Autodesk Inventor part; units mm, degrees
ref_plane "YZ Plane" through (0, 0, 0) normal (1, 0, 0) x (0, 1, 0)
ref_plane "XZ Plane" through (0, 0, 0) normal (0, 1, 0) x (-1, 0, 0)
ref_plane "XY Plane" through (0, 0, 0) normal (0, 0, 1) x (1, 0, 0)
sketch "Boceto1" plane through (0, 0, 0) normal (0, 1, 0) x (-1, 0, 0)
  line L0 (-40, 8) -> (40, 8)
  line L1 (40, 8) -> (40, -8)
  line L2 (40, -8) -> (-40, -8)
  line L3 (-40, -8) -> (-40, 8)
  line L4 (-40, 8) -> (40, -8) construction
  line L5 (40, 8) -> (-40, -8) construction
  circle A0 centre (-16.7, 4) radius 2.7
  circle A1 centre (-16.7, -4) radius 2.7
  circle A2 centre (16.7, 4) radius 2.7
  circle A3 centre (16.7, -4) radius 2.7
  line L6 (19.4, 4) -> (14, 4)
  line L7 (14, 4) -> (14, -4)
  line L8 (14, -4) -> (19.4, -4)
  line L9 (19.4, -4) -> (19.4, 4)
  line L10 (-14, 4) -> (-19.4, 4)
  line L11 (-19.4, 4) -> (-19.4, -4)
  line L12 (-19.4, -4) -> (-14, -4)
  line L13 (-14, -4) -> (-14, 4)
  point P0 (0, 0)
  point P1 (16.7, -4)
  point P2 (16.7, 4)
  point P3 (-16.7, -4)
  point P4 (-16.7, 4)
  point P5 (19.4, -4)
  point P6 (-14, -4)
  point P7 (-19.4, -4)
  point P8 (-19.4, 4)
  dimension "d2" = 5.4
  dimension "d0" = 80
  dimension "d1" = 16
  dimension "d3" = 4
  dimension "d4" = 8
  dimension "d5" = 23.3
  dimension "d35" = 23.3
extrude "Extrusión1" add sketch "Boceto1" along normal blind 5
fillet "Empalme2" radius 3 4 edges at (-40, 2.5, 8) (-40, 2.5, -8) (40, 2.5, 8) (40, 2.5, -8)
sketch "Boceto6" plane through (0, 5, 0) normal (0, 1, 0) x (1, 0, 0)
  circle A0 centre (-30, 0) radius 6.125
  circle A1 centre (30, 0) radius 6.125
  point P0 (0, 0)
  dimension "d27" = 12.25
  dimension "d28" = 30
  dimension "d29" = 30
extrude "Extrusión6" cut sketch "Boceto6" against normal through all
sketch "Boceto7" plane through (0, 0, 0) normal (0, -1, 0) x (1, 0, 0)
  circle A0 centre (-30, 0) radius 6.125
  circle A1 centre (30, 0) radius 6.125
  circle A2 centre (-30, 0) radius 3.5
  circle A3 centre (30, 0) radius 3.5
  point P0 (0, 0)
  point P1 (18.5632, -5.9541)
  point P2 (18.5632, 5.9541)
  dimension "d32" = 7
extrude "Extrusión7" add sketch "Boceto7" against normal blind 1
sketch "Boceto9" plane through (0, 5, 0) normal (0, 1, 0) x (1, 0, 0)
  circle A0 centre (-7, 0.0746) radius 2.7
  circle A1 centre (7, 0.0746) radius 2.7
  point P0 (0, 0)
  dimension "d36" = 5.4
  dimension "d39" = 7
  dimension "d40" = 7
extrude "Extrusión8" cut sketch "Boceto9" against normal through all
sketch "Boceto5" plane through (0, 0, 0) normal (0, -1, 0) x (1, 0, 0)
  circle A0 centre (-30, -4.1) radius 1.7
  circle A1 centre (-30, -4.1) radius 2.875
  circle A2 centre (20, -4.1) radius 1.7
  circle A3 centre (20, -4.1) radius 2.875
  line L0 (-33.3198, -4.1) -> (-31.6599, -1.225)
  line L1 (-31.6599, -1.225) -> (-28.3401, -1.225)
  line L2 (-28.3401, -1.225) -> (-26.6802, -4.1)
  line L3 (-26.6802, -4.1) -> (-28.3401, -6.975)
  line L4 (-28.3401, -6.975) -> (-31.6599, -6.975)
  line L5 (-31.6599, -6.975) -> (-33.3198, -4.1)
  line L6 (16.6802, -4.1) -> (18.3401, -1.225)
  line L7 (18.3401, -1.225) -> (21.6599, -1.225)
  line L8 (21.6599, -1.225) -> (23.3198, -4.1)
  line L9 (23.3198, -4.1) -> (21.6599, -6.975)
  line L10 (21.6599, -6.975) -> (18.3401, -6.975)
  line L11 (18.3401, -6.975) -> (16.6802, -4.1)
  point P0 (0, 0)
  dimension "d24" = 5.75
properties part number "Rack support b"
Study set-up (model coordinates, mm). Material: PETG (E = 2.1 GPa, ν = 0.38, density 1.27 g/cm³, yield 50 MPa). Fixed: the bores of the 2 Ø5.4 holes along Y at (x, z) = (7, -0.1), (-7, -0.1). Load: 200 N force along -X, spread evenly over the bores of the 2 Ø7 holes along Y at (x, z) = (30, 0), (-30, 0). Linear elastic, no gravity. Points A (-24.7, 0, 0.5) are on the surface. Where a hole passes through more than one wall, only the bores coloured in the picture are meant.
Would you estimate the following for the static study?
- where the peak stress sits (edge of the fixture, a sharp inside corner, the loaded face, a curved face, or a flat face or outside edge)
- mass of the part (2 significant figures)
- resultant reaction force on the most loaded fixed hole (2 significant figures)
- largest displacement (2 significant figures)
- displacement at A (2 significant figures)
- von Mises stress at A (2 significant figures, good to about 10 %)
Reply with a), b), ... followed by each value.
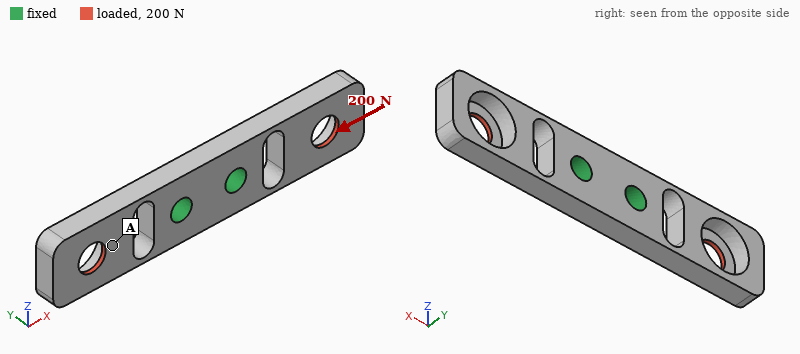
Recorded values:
a) a curved face
b) 5.7 g
c) 100 N
d) 0.81 mm
e) 0.30 mm
f) 3.6 MPa
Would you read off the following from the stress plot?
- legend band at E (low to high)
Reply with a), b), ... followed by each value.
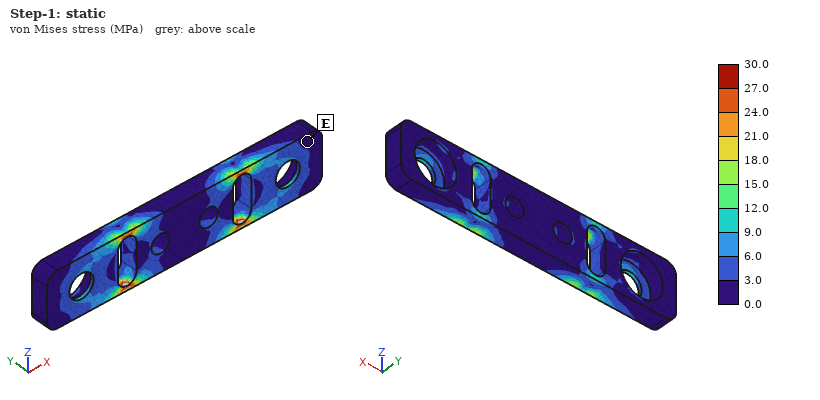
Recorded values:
a) 0.0 to 3.0 MPa
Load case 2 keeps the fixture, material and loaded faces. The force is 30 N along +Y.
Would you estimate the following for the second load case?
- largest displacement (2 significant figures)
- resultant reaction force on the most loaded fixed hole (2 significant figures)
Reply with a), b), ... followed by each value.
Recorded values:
a) 0.82 mm
b) 15 N
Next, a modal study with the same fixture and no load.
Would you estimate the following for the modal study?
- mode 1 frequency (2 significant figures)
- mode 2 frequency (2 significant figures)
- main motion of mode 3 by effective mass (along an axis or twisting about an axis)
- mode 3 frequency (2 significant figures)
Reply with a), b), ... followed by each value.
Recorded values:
a) 690 Hz
b) 690 Hz
c) twisting about Y
d) 1700 Hz
